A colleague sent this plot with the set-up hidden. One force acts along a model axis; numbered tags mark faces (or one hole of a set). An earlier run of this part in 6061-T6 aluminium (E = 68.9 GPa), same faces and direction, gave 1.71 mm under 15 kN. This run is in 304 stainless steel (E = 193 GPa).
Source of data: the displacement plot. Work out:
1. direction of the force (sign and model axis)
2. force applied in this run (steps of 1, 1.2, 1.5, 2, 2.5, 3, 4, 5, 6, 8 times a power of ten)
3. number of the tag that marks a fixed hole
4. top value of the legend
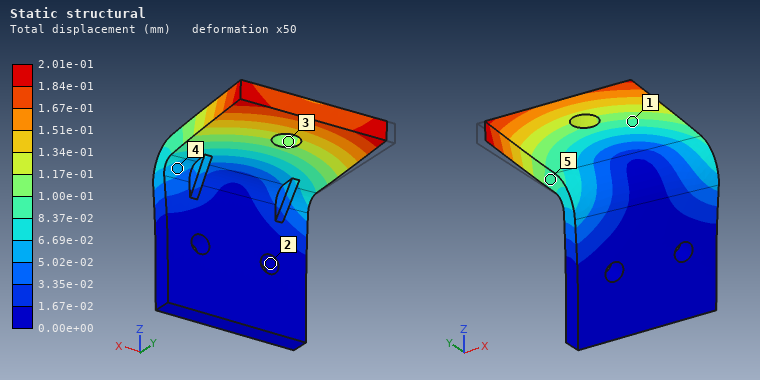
+X
5 kN
2
2.01e-01 mm
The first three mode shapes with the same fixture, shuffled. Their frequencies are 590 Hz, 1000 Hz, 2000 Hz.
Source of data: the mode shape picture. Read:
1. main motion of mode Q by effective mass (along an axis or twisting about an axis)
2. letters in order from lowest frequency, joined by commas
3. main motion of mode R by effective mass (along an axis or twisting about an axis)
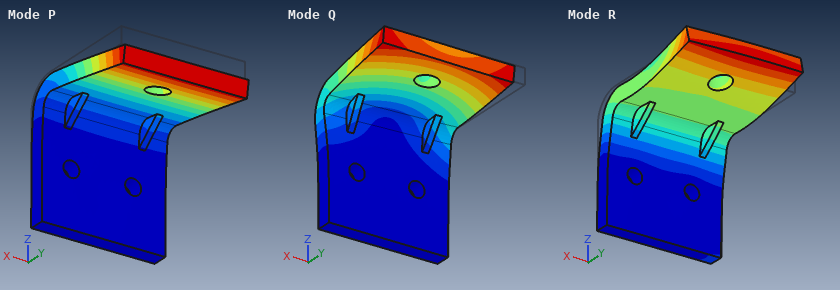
along X
P, Q, R
along Y
